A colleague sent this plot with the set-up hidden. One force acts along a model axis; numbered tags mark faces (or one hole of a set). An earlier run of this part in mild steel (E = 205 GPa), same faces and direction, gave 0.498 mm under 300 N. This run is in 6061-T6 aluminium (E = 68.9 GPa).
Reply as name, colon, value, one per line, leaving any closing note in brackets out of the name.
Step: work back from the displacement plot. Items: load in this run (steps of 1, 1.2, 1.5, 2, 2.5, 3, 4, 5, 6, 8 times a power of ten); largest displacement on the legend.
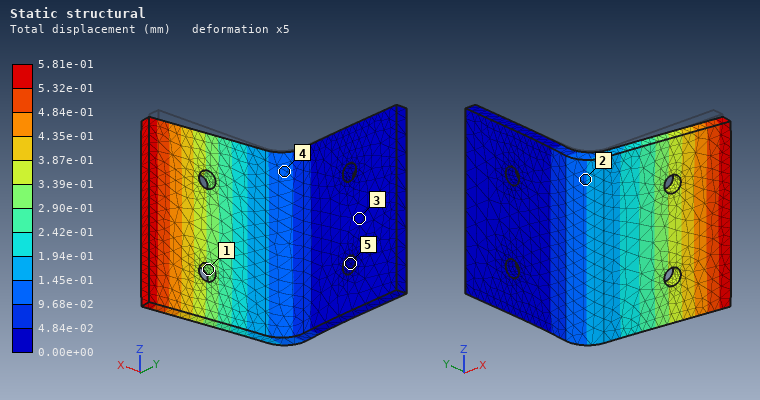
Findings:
load in this run: 120 N
largest displacement on the legend: 5.81e-01 mm
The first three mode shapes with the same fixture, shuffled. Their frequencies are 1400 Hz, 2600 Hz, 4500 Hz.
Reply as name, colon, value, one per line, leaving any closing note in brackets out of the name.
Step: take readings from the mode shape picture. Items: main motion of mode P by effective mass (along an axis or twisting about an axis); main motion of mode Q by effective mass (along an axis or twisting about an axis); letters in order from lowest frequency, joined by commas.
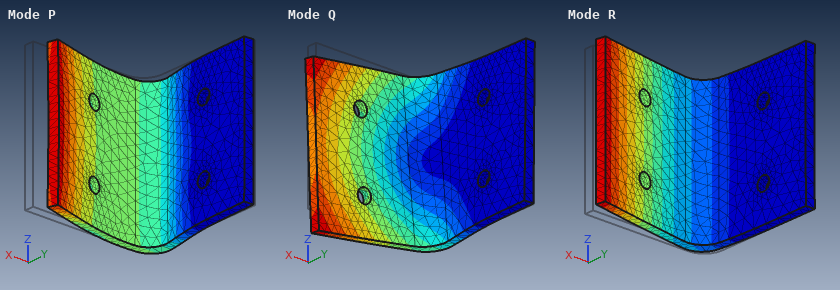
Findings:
main motion of mode P by effective mass: along X
main motion of mode Q by effective mass: along Z
letters in order from lowest frequency, joined by commas: R, Q, P
